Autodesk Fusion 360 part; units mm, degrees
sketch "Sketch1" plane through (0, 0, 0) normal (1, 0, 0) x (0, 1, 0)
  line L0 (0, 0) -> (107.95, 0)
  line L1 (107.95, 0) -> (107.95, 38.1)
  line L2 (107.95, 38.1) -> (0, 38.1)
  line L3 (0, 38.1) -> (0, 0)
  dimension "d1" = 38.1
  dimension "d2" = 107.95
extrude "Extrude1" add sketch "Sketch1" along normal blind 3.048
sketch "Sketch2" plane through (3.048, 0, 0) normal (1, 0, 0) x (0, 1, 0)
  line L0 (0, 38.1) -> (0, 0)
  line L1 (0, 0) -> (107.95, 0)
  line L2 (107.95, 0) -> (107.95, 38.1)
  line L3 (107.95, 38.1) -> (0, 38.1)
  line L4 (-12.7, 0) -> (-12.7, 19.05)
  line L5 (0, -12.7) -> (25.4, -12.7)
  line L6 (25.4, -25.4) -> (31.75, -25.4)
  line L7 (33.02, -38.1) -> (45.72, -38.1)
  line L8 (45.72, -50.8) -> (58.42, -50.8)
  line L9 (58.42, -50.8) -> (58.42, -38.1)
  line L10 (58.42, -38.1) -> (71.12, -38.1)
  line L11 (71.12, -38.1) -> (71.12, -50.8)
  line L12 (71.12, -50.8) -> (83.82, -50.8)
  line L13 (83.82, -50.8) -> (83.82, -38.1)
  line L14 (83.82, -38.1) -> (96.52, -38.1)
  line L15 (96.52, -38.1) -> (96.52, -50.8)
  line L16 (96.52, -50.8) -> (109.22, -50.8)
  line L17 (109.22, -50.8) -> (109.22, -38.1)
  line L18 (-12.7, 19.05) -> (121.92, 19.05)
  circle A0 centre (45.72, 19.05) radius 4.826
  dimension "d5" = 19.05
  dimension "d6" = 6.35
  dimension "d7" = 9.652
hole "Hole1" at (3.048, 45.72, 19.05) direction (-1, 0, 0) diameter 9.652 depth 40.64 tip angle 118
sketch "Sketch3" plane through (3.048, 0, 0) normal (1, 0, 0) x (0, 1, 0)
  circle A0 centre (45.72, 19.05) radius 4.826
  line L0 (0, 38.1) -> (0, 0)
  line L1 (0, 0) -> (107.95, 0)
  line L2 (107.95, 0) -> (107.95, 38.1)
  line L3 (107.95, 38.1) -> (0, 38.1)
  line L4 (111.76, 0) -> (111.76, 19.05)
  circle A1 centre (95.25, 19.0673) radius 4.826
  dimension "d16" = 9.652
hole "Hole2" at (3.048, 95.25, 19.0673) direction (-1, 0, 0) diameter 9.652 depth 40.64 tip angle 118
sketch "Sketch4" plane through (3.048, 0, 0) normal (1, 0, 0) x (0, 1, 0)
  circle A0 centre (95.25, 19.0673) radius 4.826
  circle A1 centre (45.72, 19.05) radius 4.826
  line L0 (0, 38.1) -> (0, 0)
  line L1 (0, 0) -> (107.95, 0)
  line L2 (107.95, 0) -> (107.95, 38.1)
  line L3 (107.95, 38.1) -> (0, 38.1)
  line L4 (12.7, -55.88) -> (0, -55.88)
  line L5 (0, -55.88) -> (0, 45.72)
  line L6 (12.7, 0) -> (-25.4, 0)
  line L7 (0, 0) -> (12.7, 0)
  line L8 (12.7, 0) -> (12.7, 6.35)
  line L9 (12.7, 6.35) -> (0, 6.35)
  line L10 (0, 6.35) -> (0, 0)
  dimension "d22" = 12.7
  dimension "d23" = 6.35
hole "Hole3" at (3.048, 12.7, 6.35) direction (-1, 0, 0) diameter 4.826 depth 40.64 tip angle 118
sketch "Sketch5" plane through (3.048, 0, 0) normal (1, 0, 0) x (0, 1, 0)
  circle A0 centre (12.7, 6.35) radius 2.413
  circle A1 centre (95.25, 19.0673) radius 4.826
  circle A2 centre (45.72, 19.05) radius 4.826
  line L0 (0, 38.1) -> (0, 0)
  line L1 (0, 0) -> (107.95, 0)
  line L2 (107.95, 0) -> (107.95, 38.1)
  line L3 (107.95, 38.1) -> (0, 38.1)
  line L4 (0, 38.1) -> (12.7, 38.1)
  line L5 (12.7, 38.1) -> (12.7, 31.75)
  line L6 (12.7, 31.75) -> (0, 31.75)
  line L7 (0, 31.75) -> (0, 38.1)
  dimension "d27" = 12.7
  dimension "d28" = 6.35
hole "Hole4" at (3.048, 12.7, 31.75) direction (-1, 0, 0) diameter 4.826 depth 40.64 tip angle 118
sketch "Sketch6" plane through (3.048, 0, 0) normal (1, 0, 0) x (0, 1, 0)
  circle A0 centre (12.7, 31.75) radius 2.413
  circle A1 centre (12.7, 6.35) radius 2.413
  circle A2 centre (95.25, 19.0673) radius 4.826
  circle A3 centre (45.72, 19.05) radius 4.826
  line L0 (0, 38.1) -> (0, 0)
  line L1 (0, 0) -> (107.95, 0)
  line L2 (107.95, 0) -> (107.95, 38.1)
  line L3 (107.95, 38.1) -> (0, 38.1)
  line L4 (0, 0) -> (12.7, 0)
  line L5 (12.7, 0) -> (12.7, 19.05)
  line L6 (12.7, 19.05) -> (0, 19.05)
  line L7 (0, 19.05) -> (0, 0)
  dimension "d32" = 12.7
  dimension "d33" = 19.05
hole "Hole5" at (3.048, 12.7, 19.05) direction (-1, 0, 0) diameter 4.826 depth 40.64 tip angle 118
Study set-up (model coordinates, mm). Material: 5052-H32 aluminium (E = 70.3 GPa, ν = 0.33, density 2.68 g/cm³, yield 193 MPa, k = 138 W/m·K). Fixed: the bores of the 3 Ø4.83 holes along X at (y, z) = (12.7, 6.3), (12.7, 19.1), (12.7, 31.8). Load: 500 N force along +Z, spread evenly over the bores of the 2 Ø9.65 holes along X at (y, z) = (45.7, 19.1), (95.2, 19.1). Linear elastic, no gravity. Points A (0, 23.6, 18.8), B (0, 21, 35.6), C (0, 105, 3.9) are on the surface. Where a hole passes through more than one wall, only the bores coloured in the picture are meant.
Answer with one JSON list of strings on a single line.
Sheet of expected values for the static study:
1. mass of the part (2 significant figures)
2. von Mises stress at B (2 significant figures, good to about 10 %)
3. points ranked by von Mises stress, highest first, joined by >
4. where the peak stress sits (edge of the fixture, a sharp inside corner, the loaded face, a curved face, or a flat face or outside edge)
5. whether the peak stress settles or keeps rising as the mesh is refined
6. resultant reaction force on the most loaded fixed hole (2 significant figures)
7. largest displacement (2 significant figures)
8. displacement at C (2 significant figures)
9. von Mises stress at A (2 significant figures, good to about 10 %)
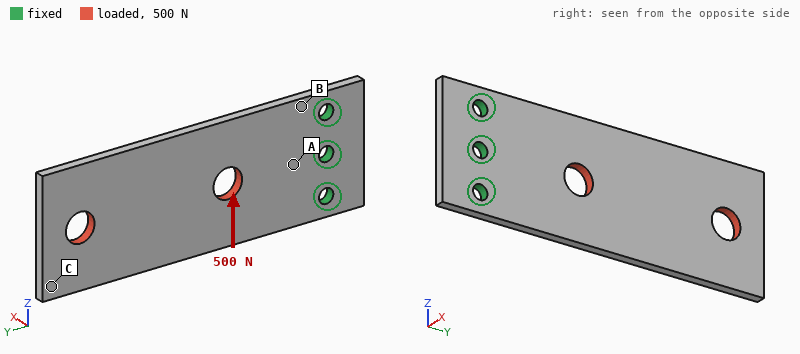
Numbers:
["32 g", "28 MPa", "B > A > C", "edge of the fixture", "keeps rising", "1.0 kN", "87 µm", "83 µm", "12 MPa"]
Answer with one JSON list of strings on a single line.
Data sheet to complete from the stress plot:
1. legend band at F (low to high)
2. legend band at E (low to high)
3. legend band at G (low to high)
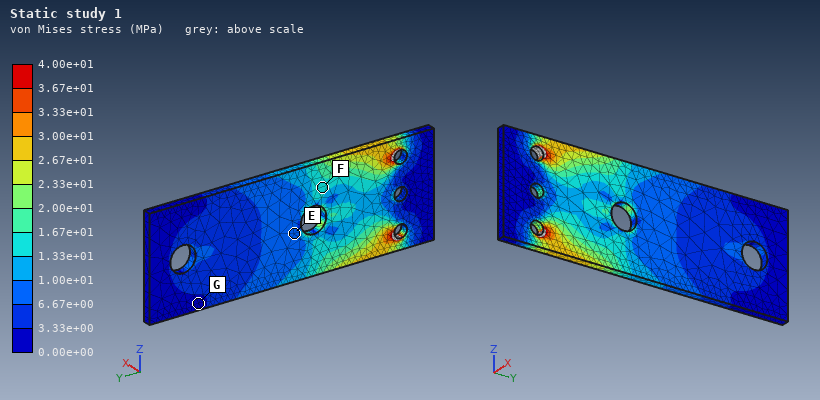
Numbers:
["1.33e+01 to 1.67e+01 MPa", "6.67e+00 to 1.00e+01 MPa", "0.00e+00 to 3.33e+00 MPa"]
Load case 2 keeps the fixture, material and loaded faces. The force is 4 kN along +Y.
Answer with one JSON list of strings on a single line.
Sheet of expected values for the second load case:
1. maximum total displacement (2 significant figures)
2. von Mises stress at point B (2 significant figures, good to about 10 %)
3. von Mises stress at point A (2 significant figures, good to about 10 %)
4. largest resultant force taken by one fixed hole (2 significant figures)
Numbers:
["37 µm", "33 MPa", "34 MPa", "1.4 kN"]
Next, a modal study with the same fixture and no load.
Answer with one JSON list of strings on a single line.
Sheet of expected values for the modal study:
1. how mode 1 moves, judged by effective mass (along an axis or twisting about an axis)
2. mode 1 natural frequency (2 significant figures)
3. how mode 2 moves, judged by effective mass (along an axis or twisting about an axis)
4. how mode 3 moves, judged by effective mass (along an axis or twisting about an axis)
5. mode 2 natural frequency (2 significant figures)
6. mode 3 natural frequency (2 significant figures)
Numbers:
["along X", "290 Hz", "twisting about Y", "along X", "1400 Hz", "1800 Hz"]
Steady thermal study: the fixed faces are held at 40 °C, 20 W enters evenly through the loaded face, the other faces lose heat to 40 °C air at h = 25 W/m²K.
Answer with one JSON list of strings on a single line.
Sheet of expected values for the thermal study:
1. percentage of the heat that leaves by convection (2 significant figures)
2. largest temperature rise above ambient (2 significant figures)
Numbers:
["31 %", "55 K"]
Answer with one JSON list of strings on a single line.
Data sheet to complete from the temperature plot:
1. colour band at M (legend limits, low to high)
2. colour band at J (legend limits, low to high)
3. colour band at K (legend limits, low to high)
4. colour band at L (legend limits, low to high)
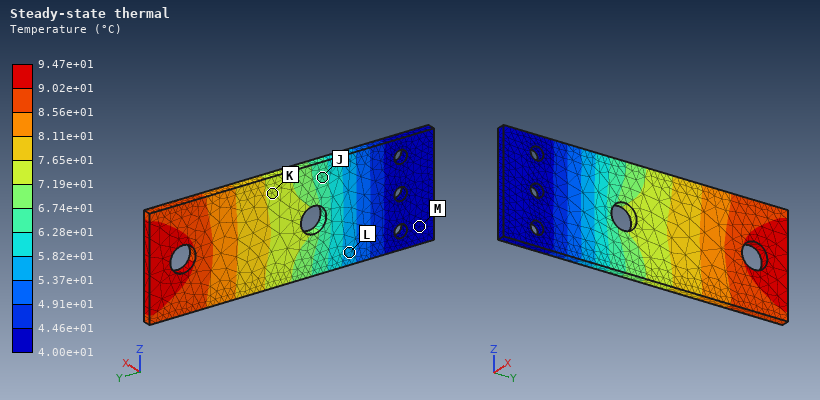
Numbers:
["4.00e+01 to 4.46e+01 °C", "6.28e+01 to 6.74e+01 °C", "7.19e+01 to 7.65e+01 °C", "5.37e+01 to 5.82e+01 °C"]
